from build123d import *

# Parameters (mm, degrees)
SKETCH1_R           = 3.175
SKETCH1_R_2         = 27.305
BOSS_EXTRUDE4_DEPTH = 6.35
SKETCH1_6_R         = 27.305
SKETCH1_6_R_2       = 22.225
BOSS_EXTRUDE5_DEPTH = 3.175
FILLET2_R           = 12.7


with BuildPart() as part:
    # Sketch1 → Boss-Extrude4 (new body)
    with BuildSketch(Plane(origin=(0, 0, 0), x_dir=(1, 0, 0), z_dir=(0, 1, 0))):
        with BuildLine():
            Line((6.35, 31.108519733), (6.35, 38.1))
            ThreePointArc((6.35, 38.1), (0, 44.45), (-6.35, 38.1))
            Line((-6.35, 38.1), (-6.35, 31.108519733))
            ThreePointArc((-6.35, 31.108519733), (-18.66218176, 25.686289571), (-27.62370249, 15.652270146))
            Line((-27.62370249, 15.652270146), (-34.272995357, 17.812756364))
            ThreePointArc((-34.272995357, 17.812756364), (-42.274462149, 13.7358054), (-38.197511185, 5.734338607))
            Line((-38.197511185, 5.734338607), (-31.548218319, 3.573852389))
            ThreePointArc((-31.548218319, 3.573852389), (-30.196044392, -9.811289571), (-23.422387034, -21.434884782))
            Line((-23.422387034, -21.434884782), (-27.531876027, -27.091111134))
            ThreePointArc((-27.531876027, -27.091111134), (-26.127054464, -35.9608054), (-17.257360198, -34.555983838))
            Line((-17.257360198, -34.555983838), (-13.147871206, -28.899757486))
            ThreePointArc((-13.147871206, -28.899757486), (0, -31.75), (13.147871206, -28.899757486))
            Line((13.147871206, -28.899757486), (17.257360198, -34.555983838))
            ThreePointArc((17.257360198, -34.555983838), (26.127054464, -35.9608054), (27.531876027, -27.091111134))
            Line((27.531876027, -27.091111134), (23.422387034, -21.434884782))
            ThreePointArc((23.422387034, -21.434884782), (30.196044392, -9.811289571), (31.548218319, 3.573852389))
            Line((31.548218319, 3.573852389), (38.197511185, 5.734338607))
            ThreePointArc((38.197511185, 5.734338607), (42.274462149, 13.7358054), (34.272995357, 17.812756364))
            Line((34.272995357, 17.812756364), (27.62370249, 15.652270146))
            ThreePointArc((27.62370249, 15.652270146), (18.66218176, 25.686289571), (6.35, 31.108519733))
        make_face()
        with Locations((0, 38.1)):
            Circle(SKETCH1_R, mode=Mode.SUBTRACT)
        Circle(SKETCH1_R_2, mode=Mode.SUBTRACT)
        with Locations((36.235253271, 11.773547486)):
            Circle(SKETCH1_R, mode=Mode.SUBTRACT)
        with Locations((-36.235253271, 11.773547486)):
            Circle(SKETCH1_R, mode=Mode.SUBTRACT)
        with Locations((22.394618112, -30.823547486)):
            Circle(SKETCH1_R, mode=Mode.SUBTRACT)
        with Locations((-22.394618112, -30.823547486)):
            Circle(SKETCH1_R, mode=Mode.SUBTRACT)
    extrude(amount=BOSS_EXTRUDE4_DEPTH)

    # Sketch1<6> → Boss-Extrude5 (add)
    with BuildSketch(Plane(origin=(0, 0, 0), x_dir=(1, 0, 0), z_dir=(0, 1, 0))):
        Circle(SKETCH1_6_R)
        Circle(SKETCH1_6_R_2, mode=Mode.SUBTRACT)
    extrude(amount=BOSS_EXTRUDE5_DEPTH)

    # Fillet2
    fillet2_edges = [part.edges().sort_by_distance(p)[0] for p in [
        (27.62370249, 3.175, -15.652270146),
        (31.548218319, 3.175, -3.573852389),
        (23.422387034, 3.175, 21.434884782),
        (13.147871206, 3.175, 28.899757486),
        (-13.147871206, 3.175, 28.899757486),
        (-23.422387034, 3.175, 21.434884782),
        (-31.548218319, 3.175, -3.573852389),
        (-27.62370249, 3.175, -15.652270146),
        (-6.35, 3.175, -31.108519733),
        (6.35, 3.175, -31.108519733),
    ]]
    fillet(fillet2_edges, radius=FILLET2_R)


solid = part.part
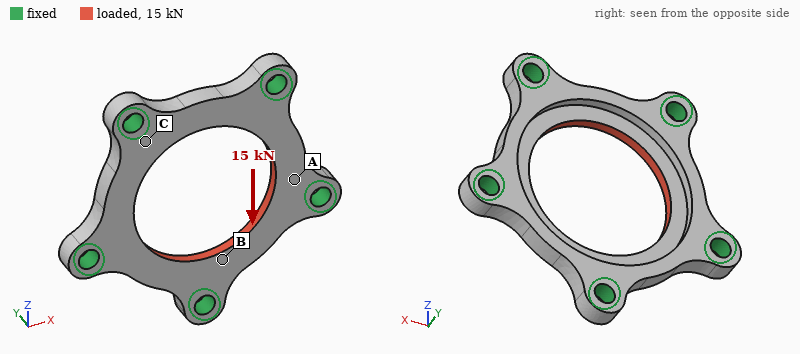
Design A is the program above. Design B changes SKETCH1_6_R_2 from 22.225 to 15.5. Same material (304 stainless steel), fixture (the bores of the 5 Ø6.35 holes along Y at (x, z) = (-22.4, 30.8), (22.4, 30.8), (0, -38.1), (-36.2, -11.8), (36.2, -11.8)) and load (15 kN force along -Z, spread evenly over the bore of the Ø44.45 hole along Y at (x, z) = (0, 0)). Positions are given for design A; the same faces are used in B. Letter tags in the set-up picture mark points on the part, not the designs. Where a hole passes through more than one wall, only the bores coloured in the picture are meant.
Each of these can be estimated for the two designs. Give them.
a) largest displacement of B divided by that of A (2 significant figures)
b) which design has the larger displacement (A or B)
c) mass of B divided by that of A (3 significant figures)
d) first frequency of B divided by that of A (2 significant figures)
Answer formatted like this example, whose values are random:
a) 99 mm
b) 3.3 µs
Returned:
a) 0.88
b) A
c) 1.21
d) 0.63
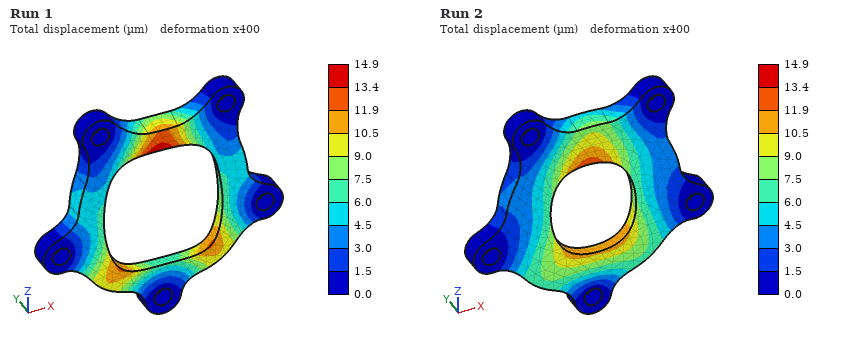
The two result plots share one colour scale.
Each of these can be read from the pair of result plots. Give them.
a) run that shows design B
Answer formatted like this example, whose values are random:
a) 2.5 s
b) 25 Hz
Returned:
a) Run 2
